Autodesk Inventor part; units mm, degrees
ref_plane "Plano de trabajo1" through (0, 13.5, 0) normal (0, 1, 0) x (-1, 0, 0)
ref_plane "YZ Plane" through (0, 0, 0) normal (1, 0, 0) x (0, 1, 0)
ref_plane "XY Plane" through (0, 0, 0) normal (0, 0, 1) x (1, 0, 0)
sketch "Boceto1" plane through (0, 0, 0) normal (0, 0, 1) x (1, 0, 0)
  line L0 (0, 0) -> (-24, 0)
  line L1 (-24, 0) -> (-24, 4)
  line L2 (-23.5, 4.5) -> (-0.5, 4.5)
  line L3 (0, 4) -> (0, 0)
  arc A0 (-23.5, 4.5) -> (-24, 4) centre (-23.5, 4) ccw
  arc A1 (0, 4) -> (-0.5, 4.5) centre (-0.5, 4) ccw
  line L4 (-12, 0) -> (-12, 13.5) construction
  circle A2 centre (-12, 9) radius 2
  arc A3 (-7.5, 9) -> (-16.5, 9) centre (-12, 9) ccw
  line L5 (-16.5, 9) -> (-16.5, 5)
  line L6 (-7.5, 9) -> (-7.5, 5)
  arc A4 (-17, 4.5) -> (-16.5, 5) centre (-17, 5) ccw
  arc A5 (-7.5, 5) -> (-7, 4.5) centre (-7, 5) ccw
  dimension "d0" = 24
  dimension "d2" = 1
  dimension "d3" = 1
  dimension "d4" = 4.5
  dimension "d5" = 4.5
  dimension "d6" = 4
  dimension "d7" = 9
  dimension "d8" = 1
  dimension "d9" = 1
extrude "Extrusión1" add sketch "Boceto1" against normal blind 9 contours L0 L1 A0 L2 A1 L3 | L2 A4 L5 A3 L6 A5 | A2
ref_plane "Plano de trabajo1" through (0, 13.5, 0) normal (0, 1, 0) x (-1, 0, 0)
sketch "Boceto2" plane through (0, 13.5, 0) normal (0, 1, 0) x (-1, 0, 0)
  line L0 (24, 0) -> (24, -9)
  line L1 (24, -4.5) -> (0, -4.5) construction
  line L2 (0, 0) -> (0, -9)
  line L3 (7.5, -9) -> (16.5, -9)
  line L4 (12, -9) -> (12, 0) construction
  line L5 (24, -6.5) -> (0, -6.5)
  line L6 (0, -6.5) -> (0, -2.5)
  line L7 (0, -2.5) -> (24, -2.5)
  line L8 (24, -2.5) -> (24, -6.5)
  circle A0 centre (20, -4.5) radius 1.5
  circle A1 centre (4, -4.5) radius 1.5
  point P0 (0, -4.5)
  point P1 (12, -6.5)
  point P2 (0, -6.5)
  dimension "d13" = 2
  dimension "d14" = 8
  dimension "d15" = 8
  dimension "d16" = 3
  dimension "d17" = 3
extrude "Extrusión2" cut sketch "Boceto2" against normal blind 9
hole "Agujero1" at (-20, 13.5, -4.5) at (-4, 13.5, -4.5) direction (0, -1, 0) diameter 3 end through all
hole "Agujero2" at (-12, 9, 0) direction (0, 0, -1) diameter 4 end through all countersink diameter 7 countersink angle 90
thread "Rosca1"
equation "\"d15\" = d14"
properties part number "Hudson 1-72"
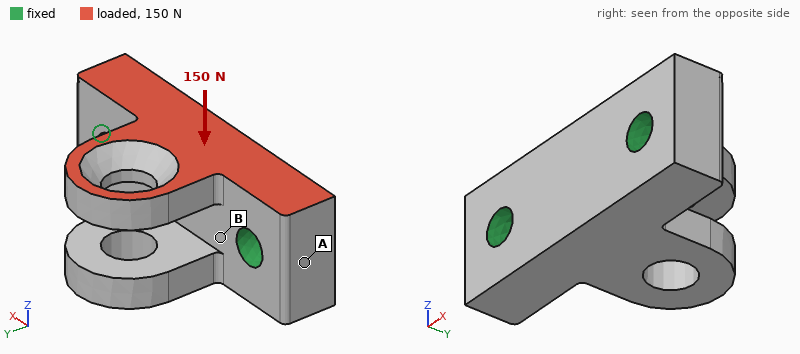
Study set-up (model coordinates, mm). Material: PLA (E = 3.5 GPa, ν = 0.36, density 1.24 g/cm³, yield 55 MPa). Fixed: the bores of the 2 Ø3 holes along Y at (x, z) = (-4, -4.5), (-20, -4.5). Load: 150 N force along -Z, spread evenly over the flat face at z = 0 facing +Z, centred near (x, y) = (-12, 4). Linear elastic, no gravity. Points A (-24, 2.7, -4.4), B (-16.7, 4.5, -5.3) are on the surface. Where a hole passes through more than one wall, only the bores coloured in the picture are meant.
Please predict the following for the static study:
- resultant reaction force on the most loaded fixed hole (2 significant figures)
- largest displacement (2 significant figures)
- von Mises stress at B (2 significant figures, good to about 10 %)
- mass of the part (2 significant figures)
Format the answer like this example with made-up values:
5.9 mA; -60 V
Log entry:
76 N; 0.18 mm; 4.3 MPa; 1.5 g
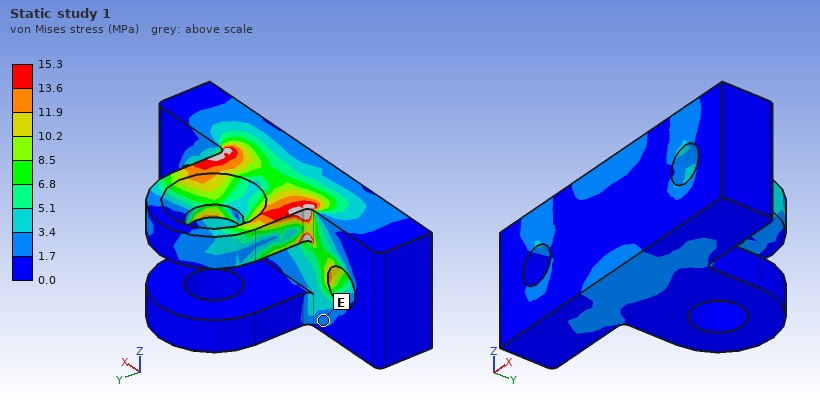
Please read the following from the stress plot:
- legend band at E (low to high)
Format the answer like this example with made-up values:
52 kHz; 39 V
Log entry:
1.7 to 3.4 MPa
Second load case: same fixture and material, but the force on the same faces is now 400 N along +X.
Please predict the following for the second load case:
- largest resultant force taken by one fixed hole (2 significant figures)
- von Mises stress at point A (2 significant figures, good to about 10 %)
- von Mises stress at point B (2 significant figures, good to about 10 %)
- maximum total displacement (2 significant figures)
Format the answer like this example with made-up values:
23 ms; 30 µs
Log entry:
220 N; 5.4 MPa; 4.1 MPa; 0.13 mm
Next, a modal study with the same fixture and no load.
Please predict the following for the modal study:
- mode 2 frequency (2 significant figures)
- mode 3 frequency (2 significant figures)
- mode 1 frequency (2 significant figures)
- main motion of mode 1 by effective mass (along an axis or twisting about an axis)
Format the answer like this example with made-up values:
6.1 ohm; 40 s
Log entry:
7300 Hz; 14 kHz; 6600 Hz; along Z
